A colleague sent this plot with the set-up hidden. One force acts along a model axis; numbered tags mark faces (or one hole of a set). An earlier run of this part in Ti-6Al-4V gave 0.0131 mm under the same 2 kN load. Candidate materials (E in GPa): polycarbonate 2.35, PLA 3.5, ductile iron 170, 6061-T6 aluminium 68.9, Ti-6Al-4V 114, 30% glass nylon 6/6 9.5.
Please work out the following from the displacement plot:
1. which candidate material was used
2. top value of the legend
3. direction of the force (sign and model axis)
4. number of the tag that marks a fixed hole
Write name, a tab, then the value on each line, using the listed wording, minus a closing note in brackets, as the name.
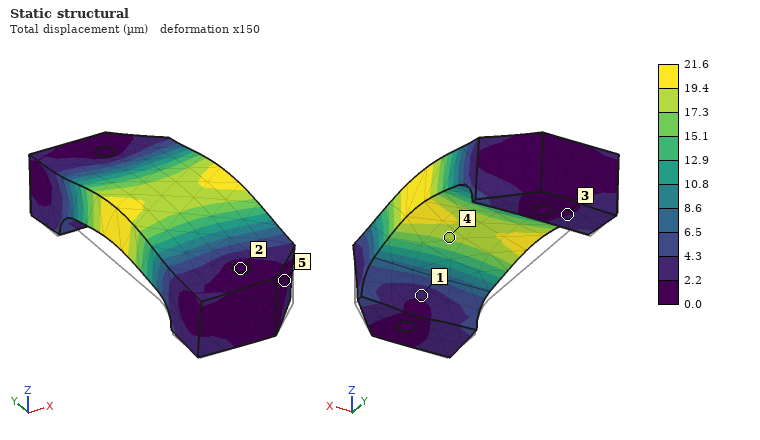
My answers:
which candidate material was used	6061-T6 aluminium
top value of the legend	21.6 µm
direction of the force	+Z
number of the tag that marks a fixed hole	2
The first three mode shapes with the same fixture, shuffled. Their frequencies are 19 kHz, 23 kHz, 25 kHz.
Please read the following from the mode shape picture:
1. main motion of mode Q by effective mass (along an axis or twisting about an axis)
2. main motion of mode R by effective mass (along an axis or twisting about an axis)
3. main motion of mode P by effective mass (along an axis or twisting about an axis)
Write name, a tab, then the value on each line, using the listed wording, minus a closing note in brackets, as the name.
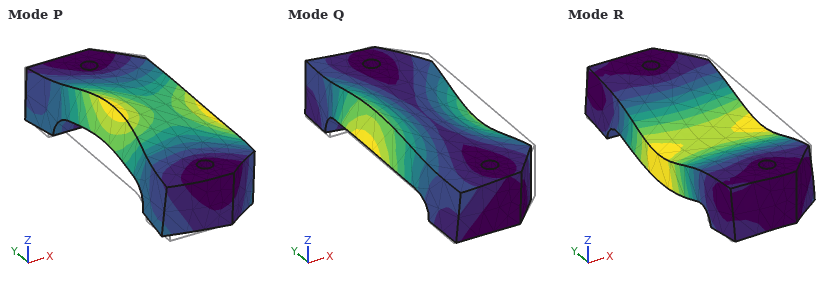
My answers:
main motion of mode Q by effective mass	along X
main motion of mode R by effective mass	along Z
main motion of mode P by effective mass	along X
